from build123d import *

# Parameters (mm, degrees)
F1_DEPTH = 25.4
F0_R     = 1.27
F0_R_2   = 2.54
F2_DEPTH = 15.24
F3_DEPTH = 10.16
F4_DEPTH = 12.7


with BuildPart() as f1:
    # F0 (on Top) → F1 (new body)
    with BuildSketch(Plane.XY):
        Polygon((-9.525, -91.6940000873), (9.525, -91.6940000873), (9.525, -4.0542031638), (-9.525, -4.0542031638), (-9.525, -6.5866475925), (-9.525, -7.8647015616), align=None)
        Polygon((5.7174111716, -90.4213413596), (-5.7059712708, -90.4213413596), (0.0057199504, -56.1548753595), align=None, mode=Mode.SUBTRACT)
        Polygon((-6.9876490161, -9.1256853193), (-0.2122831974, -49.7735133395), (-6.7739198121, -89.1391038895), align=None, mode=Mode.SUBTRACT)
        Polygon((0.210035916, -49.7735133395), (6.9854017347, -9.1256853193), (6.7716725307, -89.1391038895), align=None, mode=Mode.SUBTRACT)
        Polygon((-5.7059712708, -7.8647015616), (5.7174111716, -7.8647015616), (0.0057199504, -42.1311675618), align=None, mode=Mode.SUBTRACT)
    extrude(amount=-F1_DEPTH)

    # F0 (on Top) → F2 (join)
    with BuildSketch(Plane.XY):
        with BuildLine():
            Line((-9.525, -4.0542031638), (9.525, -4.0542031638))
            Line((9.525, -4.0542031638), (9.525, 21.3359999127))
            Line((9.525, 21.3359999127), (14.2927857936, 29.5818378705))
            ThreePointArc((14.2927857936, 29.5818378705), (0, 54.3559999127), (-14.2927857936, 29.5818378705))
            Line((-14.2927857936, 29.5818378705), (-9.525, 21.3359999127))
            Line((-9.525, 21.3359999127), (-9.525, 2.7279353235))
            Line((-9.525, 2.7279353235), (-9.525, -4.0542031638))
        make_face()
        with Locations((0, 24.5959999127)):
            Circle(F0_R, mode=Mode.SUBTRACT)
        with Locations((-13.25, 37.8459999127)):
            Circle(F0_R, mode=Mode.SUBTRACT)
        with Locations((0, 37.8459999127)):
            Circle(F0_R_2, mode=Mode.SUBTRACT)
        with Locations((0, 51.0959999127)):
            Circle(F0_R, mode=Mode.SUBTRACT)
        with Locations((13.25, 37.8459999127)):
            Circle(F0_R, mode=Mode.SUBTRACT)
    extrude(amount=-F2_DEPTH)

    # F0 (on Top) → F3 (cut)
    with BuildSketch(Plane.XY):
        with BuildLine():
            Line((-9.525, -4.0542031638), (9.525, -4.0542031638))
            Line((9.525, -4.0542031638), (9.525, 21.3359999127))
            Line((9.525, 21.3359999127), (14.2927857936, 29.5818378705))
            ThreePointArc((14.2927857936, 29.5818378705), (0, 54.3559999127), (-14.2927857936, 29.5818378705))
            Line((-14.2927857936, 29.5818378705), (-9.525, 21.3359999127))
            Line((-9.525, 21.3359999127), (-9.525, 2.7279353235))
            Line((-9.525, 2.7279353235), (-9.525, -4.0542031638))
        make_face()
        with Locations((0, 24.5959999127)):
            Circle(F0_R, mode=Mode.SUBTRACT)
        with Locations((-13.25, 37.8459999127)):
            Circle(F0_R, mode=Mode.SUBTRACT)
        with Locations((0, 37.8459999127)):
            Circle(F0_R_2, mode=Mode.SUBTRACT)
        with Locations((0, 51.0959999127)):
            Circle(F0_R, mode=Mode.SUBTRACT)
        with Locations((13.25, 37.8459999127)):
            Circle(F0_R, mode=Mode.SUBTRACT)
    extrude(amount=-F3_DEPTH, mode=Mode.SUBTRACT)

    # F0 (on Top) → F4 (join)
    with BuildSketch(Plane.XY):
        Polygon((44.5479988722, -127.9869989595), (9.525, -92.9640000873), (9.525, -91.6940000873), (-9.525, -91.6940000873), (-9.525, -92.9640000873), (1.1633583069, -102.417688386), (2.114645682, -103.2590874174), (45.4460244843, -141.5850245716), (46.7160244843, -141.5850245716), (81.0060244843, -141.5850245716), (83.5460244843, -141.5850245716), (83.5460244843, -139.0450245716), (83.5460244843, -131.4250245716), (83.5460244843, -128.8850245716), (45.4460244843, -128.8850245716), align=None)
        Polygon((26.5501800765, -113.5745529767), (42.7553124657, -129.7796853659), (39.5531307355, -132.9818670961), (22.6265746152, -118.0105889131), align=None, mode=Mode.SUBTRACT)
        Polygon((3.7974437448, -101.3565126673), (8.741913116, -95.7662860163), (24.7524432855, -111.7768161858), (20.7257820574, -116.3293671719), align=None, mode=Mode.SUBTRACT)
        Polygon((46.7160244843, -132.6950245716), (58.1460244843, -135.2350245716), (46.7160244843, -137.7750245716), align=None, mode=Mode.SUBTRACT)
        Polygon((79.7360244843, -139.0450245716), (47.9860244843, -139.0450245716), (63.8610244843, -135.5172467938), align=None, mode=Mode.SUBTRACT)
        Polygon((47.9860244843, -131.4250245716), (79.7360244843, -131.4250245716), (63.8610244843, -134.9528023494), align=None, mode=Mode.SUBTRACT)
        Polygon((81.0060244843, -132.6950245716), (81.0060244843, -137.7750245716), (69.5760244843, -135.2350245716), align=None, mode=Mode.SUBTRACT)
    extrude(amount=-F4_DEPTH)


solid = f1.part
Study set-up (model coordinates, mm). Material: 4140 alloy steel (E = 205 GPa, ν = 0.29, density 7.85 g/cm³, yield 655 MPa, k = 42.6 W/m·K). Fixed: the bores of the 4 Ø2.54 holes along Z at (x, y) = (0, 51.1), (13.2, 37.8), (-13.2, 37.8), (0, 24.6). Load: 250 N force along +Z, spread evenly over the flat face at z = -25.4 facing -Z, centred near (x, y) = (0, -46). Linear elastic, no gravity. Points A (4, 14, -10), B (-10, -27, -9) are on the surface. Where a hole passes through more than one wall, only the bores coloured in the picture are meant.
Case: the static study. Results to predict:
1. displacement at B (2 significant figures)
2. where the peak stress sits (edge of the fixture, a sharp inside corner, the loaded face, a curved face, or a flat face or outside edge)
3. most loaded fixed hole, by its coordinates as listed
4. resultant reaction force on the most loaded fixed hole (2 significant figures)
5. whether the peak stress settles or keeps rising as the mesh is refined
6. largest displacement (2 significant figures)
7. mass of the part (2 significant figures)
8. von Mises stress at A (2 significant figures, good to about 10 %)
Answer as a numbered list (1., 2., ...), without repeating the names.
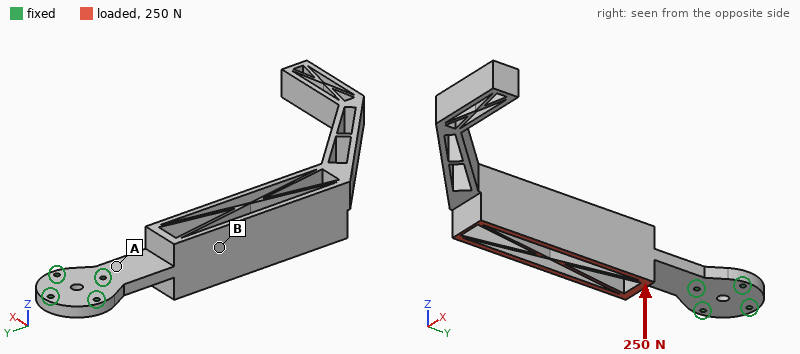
1. 0.39 mm
2. edge of the fixture
3. (0, 24.6)
4. 890 N
5. keeps rising
6. 1.6 mm
7. 280 g
8. 180 MPa
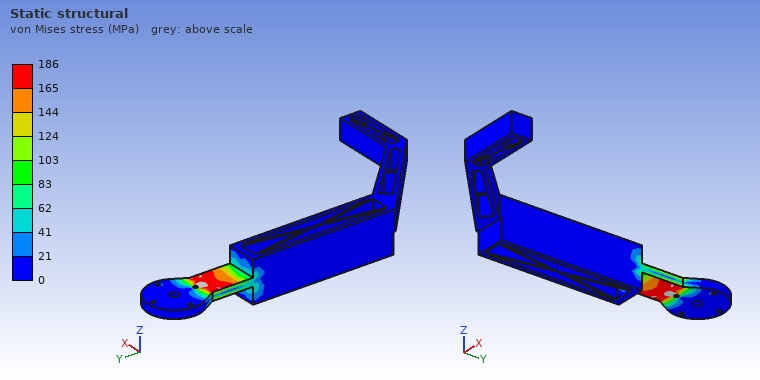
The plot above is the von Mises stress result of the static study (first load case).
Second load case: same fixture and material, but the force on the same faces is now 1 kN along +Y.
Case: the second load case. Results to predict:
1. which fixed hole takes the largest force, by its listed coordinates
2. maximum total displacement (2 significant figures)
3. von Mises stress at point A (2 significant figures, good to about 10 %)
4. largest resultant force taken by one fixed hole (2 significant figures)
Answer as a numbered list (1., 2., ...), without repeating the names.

1. (0, 24.6)
2. 1.4 mm
3. 140 MPa
4. 820 N
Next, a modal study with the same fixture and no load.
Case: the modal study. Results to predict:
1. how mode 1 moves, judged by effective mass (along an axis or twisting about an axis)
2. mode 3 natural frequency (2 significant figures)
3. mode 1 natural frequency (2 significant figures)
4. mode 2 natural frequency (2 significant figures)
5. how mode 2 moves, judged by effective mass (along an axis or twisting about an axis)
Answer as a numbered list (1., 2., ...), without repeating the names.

1. along Z
2. 460 Hz
3. 130 Hz
4. 350 Hz
5. along X
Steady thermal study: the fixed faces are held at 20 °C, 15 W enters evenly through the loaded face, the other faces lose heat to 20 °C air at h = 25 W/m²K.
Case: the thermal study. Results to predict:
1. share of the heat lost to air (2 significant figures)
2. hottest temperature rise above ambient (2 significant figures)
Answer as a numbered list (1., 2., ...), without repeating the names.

1. 84 %
2. 32 K
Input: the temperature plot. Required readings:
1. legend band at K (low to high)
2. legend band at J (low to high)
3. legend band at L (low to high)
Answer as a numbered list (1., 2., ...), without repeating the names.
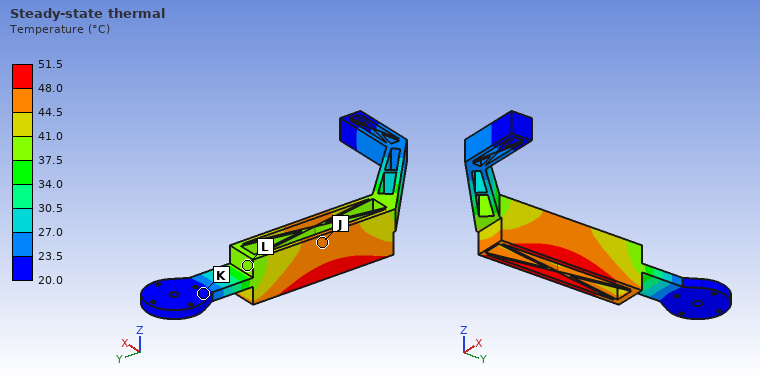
1. 20.0 to 23.5 °C
2. 44.5 to 48.0 °C
3. 37.5 to 41.0 °C
